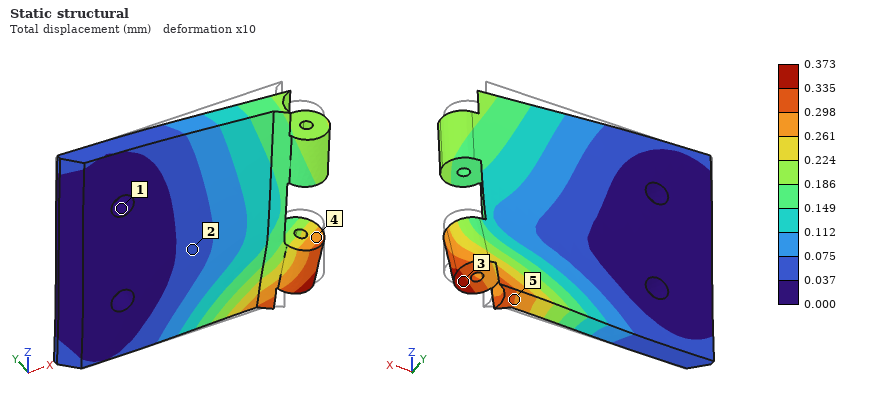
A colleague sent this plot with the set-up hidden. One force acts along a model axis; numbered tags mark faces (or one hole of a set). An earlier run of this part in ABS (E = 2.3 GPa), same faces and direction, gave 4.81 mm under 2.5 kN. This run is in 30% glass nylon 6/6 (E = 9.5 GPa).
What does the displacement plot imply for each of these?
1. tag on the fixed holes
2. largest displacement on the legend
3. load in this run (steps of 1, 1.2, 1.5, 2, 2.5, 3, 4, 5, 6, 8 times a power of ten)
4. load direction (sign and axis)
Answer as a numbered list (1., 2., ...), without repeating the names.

1. 1
2. 0.373 mm
3. 800 N
4. -Z
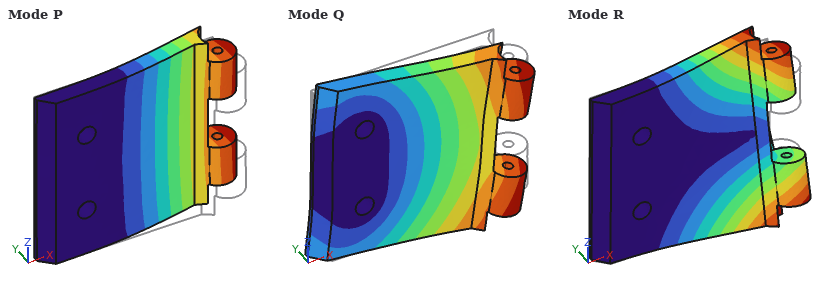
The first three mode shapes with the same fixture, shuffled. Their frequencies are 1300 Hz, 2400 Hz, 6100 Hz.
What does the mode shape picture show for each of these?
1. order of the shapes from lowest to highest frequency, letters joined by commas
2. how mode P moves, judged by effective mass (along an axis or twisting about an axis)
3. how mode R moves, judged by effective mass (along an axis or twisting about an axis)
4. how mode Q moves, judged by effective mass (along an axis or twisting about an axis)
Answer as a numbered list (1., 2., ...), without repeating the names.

1. P, R, Q
2. along Y
3. twisting about X
4. along Z
